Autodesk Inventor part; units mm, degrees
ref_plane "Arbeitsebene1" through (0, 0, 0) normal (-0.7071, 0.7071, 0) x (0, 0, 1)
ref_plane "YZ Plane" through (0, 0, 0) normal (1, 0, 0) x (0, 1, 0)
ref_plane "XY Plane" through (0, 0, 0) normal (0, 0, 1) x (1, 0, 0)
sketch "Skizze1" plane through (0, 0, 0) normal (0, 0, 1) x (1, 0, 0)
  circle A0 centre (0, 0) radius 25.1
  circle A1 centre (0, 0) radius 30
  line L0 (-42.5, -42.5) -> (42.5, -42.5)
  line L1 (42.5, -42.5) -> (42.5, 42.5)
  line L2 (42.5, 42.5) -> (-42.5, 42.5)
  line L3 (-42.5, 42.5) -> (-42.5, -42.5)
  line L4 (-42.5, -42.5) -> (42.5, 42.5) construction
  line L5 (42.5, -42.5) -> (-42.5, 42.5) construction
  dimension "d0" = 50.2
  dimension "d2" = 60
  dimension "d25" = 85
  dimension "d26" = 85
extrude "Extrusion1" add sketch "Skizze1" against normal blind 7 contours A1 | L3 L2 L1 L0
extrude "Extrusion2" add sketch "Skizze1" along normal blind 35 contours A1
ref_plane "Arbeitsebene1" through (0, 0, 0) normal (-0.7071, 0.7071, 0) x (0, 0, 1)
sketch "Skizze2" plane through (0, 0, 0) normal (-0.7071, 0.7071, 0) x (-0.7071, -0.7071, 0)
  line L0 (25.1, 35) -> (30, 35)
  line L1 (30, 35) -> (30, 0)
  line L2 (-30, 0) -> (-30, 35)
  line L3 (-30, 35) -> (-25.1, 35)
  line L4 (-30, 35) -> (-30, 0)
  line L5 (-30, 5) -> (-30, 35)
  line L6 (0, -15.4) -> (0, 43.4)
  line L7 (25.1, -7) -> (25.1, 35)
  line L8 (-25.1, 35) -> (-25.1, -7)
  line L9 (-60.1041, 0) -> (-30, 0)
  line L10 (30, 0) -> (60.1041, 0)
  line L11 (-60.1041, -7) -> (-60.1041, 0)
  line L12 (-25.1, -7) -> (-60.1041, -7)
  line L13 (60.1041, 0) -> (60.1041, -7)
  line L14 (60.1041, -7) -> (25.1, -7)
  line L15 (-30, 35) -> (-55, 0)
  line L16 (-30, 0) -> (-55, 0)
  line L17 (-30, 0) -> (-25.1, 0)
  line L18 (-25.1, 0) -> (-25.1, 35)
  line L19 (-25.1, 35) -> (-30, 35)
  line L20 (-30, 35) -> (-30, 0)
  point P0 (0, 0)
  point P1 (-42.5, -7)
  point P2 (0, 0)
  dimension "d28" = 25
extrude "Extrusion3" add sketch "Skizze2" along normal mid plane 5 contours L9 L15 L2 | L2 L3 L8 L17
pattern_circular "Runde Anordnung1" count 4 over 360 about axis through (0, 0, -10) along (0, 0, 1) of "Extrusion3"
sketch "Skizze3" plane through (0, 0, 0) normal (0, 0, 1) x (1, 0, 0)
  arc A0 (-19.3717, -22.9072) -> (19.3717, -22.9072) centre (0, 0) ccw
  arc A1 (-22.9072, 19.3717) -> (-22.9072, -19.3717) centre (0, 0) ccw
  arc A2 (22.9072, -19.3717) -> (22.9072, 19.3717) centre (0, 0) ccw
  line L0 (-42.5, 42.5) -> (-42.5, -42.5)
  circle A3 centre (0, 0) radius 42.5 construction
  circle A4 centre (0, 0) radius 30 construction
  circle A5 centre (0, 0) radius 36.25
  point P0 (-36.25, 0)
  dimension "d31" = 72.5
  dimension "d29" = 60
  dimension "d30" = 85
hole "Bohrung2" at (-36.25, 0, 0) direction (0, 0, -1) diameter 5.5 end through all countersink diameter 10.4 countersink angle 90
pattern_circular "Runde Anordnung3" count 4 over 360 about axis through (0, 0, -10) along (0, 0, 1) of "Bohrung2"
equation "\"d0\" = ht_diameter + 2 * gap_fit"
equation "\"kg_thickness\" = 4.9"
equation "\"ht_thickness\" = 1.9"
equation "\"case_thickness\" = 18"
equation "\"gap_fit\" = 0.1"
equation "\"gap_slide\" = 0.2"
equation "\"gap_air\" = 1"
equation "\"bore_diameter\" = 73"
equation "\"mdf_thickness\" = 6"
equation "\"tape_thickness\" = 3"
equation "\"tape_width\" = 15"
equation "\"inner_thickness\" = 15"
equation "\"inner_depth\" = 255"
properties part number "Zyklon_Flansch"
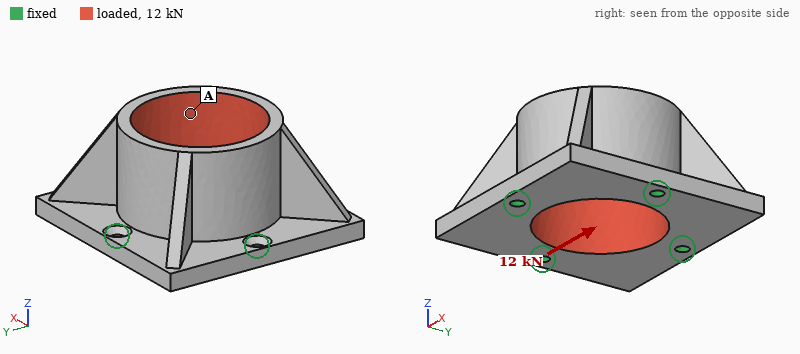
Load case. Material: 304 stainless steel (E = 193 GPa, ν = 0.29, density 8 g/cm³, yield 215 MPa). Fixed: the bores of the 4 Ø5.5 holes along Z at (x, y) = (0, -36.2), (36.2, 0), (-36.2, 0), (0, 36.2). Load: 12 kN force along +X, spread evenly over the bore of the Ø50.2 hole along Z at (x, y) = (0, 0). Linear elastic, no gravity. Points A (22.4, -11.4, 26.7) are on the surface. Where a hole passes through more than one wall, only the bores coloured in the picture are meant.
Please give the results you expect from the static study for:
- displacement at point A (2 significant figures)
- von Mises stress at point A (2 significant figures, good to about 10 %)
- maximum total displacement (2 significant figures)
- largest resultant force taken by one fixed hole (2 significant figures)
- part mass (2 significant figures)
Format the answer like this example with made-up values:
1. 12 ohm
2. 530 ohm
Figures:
1. 14 µm
2. 13 MPa
3. 17 µm
4. 4.2 kN
5. 590 g
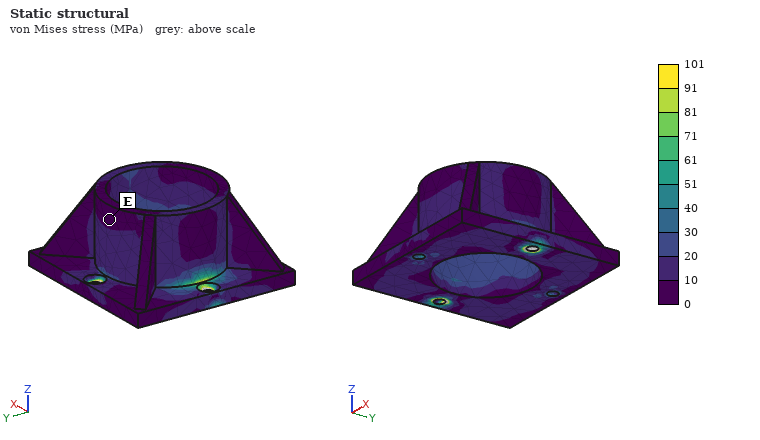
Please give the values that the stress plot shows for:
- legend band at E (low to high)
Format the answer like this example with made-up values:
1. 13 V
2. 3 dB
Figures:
1. 0 to 10 MPa
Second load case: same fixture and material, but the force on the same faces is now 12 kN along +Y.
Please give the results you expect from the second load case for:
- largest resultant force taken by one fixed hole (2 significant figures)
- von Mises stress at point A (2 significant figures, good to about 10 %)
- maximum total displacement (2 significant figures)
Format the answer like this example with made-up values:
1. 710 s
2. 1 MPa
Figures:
1. 4.2 kN
2. 12 MPa
3. 17 µm
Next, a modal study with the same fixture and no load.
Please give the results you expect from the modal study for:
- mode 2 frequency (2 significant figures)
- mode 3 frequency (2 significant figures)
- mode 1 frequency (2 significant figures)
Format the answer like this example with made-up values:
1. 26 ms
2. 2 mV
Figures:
1. 6100 Hz
2. 6100 Hz
3. 4300 Hz
